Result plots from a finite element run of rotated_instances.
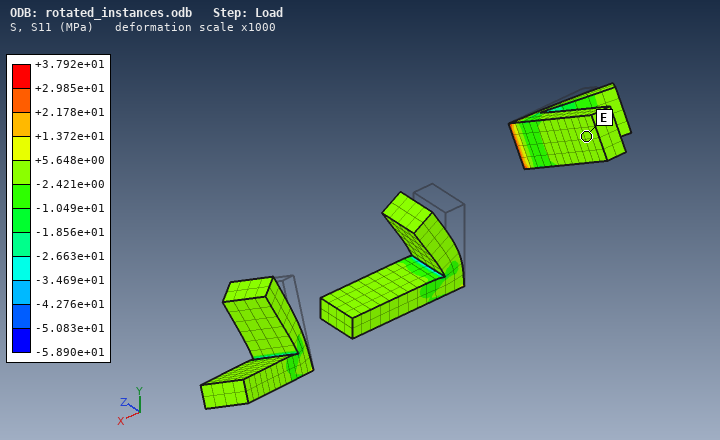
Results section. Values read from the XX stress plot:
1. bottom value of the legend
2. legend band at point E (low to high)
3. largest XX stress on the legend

-5.890e+01 MPa
-2.421e+00 to +5.648e+00 MPa
+3.792e+01 MPa
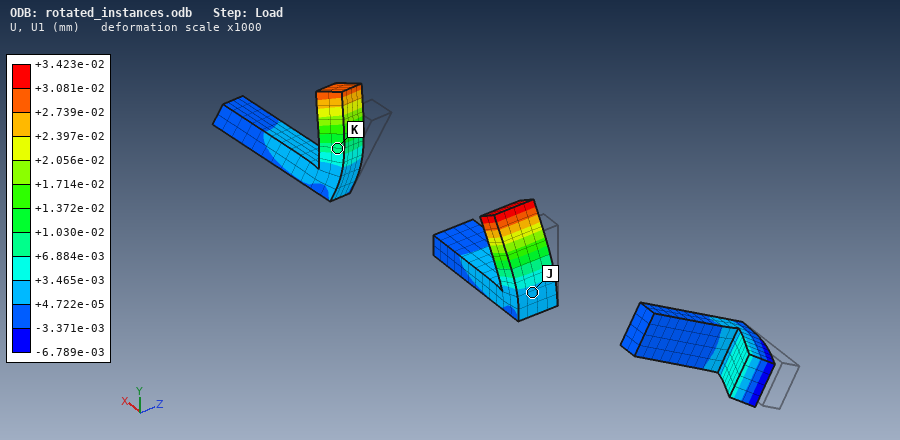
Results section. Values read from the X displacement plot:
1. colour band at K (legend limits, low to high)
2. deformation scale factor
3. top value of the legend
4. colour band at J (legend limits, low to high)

+6.884e-03 to +1.030e-02 mm
1000
+3.423e-02 mm
+4.722e-05 to +3.465e-03 mm
